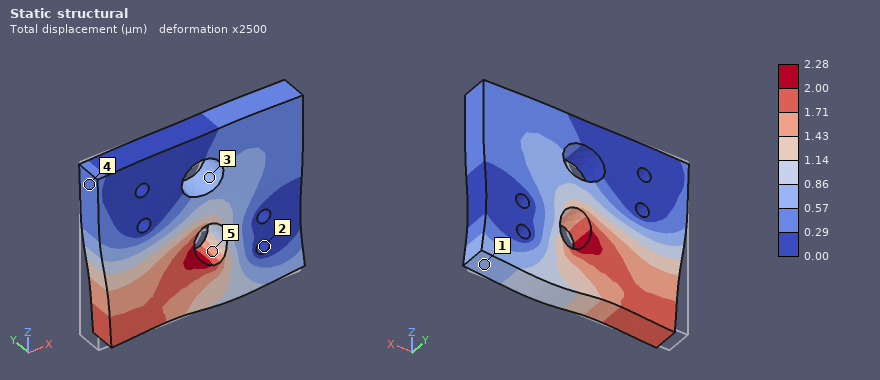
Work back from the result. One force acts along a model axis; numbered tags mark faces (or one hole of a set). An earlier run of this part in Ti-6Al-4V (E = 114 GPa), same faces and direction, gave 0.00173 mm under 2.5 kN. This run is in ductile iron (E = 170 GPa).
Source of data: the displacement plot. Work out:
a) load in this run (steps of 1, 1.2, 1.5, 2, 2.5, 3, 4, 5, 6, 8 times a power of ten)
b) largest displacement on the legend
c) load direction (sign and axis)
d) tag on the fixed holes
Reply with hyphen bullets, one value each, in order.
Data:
- 5 kN
- 2.28 µm
- +X
- 2
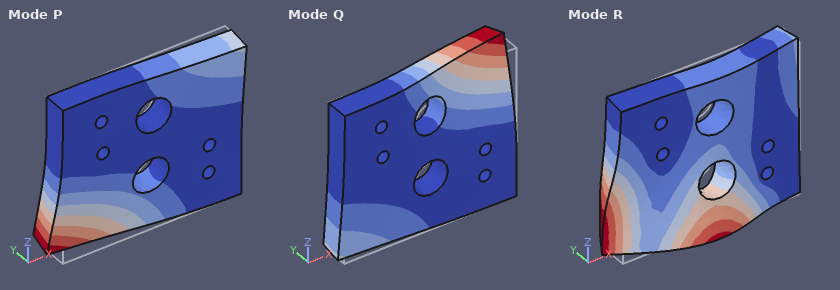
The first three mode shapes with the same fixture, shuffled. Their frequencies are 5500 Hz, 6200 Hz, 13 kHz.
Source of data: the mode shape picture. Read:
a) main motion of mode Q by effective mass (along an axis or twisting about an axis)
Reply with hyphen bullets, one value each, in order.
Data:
- along Y
